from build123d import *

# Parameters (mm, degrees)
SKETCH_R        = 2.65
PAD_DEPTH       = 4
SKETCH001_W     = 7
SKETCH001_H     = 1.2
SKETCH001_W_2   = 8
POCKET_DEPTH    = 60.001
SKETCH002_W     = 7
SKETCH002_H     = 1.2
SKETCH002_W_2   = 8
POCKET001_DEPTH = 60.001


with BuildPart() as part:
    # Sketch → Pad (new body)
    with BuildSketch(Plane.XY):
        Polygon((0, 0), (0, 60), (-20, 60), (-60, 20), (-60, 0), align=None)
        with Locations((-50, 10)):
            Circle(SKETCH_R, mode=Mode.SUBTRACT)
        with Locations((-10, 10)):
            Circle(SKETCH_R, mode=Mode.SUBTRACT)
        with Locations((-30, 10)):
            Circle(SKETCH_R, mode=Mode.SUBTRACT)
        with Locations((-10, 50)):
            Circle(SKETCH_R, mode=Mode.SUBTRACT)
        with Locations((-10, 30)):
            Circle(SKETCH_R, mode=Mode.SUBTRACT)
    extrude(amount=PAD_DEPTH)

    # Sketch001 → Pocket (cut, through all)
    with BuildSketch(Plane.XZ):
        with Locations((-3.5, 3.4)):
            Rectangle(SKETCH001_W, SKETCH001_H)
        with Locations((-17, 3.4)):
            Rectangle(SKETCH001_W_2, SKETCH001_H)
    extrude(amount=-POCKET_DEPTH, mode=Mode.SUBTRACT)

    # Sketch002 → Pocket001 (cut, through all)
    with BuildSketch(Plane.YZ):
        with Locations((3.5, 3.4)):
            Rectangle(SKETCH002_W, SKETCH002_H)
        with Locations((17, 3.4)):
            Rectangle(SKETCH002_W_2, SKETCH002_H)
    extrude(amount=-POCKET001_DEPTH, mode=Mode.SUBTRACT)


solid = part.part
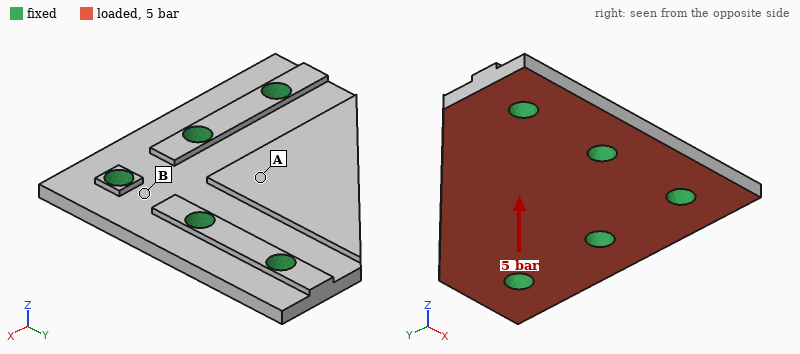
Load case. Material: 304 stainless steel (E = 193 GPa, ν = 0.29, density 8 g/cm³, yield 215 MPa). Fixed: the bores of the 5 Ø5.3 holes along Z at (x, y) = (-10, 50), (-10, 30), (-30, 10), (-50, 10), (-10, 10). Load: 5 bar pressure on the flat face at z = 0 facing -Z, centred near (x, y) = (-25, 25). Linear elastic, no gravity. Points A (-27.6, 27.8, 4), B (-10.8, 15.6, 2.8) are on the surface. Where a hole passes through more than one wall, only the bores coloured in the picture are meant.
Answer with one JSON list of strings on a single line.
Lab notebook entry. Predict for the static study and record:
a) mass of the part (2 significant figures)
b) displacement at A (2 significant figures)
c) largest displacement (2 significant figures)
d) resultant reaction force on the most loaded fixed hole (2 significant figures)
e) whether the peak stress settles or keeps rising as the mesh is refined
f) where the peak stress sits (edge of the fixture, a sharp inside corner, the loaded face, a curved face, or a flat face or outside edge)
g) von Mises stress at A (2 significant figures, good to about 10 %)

["71 g", "7.7 µm", "23 µm", "340 N", "keeps rising", "edge of the fixture", "20 MPa"]
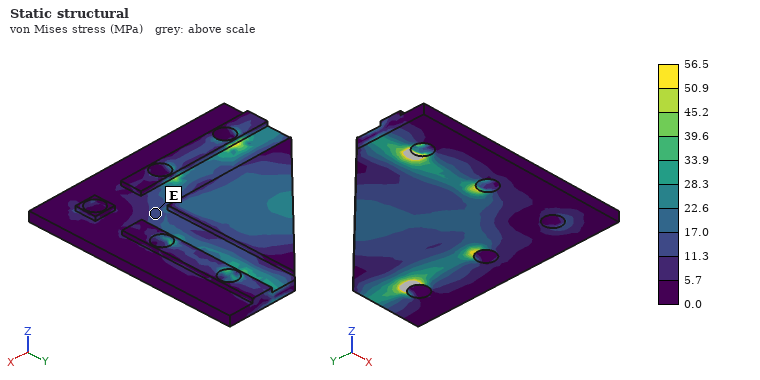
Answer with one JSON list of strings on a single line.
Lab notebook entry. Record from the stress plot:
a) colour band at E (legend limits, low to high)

["11.3 to 17.0 MPa"]
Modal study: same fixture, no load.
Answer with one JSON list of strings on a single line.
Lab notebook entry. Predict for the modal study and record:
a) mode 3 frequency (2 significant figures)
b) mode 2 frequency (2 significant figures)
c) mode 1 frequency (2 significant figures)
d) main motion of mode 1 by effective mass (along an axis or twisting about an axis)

["18 kHz", "13 kHz", "5600 Hz", "along Z"]
